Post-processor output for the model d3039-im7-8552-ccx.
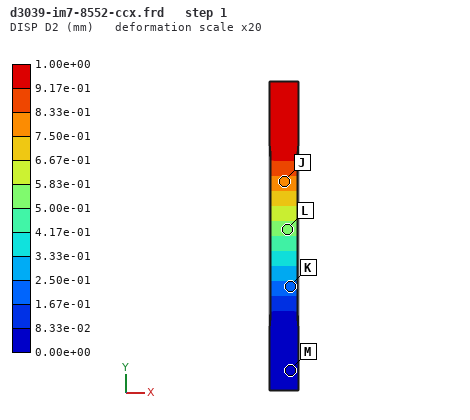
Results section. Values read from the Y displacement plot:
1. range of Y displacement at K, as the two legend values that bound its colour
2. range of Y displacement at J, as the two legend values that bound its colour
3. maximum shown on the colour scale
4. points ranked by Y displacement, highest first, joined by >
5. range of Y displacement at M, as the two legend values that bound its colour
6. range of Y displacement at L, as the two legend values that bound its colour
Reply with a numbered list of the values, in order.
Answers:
1. 1.67e-01 to 2.50e-01 mm
2. 7.50e-01 to 8.33e-01 mm
3. 1.00e+00 mm
4. J > L > K > M
5. 0.00e+00 to 8.33e-02 mm
6. 5.00e-01 to 5.83e-01 mm
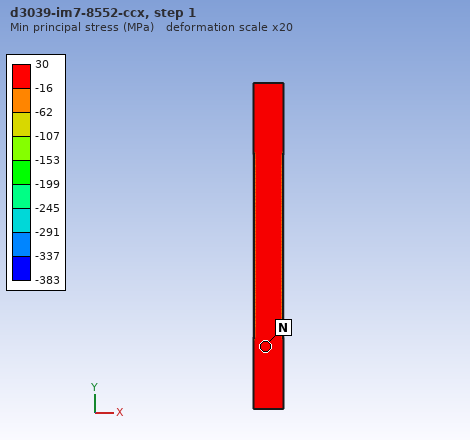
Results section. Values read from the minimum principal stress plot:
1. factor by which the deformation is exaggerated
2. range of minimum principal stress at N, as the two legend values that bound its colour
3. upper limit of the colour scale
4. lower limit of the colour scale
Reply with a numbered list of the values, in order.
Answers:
1. 20
2. -16 to 30 MPa
3. 30 MPa
4. -383 MPa
